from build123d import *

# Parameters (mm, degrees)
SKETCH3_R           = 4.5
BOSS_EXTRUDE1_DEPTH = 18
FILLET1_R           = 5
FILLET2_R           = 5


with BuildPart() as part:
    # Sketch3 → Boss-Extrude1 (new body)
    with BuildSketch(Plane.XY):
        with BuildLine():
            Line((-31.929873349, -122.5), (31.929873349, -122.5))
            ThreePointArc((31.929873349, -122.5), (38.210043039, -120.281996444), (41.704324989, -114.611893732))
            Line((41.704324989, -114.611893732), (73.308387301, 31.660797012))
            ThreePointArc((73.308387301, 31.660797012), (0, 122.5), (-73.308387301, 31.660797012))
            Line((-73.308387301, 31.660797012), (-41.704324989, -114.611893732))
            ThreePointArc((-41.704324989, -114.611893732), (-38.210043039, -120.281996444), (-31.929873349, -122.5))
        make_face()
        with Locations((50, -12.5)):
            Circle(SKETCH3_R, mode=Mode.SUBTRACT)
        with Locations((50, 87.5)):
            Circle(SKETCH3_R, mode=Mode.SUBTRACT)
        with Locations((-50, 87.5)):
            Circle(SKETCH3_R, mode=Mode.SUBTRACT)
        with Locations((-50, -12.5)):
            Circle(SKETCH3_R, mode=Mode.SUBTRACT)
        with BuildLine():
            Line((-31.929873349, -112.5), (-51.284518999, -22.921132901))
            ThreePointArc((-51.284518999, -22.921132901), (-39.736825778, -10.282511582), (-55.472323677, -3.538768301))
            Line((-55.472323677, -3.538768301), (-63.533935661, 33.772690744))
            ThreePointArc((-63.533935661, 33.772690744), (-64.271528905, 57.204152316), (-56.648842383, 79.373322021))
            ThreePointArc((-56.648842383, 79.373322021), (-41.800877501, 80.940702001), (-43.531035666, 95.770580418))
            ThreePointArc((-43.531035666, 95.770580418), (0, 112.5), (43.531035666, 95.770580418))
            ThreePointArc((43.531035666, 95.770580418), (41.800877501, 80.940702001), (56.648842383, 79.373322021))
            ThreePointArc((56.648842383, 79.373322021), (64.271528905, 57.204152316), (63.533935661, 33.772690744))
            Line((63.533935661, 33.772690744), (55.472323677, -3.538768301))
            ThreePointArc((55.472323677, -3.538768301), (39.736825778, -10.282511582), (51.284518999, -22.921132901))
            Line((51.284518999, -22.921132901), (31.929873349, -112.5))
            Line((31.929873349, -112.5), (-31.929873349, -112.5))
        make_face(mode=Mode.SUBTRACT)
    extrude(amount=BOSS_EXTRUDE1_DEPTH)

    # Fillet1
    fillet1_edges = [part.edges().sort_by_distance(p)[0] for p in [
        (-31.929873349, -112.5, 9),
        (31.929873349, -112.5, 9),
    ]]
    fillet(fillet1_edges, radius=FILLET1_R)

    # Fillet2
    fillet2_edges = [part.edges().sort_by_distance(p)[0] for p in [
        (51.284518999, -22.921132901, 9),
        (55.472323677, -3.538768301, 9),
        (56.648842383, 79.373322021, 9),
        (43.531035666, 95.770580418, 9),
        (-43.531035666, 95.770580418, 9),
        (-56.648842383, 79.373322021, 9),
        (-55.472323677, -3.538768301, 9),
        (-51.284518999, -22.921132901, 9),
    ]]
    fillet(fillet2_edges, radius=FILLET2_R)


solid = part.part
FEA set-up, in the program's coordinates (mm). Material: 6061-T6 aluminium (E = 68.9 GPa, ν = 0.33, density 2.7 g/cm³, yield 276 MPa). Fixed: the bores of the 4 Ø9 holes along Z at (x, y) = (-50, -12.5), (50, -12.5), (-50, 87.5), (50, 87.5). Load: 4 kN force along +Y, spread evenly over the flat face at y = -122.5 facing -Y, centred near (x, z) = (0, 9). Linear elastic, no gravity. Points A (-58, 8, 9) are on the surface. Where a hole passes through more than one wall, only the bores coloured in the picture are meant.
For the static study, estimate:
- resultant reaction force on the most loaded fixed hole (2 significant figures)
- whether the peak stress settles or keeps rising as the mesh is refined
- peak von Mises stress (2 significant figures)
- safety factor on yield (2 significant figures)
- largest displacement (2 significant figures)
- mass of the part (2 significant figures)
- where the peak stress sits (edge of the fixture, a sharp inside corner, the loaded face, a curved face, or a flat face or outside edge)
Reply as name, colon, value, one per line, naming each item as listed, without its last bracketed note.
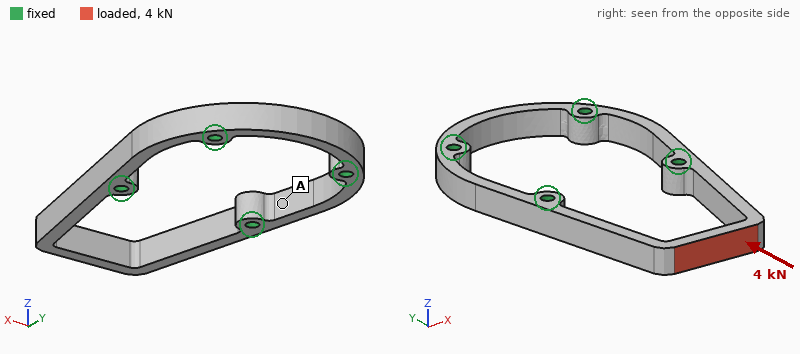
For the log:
resultant reaction force on the most loaded fixed hole: 2.0 kN
whether the peak stress settles or keeps rising as the mesh is refined: settles
peak von Mises stress: 79 MPa
safety factor on yield: 3.5
largest displacement: 0.13 mm
mass of the part: 340 g
where the peak stress sits: the loaded face
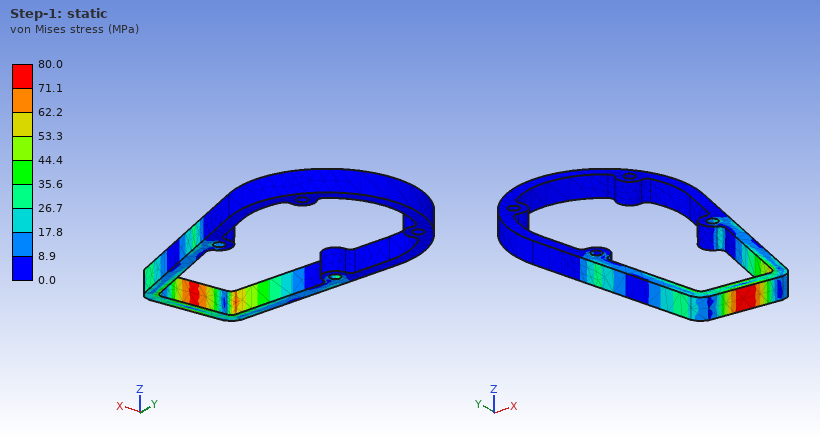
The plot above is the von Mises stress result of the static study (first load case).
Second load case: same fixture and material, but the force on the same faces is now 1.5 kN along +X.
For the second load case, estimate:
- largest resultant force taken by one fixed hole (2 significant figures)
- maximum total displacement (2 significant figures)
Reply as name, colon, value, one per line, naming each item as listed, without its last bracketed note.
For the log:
largest resultant force taken by one fixed hole: 1.0 kN
maximum total displacement: 0.44 mm
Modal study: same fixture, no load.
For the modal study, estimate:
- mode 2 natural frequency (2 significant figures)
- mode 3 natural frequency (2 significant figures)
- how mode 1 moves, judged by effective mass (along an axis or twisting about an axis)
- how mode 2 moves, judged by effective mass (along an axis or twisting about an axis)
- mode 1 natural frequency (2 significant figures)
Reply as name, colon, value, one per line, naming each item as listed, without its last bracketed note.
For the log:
mode 2 natural frequency: 1100 Hz
mode 3 natural frequency: 1900 Hz
how mode 1 moves, judged by effective mass: along Z
how mode 2 moves, judged by effective mass: along X
mode 1 natural frequency: 880 Hz
